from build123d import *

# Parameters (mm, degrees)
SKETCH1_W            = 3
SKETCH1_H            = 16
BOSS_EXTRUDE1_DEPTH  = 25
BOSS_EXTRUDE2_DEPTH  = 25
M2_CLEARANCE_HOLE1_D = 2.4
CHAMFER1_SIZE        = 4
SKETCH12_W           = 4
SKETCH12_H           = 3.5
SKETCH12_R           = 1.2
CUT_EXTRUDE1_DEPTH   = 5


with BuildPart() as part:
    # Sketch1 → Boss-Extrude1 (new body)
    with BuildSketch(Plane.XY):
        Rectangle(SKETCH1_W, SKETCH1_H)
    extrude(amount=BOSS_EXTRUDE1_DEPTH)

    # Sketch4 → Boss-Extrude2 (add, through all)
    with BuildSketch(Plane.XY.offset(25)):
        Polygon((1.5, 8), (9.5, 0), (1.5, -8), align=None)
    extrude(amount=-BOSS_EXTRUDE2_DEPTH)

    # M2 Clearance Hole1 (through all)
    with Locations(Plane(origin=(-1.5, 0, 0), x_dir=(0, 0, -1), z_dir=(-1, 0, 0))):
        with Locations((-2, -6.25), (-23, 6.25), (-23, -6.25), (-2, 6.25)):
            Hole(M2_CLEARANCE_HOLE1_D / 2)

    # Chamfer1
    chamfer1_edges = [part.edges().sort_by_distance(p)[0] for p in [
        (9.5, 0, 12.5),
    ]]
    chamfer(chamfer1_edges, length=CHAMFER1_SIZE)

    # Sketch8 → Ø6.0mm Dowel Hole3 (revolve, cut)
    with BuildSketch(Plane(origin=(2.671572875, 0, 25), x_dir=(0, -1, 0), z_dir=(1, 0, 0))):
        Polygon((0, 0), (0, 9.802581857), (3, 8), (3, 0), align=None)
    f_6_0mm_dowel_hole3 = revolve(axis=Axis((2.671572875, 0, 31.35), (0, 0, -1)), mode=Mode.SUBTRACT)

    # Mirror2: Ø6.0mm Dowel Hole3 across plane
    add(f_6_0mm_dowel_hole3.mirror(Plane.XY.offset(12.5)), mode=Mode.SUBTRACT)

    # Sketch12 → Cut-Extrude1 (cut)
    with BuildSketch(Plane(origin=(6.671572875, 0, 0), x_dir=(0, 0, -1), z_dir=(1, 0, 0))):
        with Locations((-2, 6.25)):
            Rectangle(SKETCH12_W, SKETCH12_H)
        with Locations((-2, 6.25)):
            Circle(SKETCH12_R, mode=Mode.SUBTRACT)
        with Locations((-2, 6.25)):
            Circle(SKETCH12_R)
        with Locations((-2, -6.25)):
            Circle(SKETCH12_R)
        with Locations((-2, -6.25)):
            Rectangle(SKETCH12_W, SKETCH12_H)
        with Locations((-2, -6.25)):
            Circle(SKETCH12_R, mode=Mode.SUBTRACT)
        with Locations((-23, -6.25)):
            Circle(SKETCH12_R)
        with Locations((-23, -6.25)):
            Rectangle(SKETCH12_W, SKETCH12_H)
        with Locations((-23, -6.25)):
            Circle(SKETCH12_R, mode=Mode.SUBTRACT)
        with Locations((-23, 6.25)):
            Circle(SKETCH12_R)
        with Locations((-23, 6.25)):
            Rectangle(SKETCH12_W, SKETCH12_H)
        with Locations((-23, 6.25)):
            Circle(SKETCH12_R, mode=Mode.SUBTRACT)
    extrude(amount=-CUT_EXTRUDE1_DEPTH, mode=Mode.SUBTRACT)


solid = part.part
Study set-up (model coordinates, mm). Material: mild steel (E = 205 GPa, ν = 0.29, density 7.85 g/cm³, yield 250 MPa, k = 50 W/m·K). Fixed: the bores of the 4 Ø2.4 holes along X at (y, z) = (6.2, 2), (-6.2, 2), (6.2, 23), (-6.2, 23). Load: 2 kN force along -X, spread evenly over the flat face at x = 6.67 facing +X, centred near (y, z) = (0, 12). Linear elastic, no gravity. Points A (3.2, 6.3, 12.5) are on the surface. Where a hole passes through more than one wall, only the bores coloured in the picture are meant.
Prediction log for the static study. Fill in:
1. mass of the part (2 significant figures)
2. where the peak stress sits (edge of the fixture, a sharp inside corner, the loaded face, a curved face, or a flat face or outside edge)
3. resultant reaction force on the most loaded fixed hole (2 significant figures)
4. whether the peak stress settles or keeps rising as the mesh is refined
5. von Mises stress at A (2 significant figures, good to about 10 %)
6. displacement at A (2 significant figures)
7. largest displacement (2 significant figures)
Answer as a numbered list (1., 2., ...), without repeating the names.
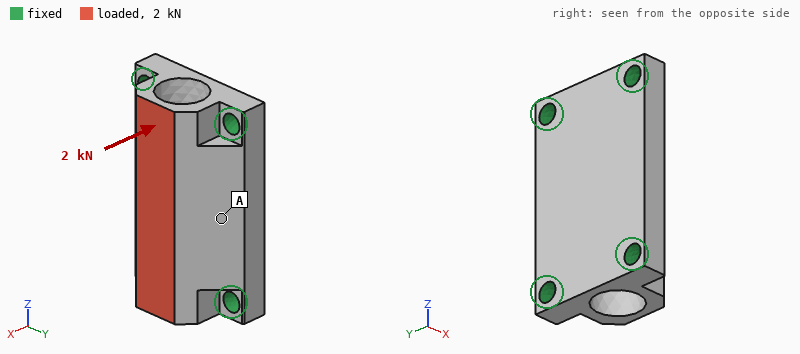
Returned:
1. 15 g
2. edge of the fixture
3. 550 N
4. keeps rising
5. 18 MPa
6. 2.2 µm
7. 3.0 µm
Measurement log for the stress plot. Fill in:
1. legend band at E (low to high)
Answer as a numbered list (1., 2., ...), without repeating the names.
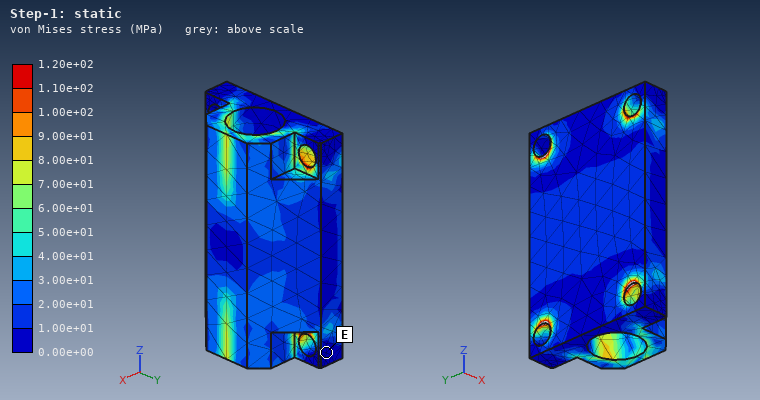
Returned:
1. 0.00e+00 to 1.00e+01 MPa
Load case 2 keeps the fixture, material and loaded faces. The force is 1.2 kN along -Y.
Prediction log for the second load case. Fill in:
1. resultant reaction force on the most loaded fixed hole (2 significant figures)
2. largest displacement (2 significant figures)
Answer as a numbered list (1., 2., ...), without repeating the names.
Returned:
1. 460 N
2. 3.6 µm
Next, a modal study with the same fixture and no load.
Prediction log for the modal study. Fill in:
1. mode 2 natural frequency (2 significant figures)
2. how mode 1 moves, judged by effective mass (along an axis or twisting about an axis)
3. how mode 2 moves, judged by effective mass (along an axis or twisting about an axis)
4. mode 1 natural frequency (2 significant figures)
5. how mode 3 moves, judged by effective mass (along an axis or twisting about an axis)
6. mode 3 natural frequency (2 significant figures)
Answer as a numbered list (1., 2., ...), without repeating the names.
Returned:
1. 43 kHz
2. along X
3. along Y
4. 39 kHz
5. along Y
6. 55 kHz
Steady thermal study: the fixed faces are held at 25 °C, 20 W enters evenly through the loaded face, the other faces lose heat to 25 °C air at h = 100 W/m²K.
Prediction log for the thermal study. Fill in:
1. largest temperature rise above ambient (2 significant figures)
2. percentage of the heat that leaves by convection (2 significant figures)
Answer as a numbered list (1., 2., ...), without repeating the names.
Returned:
1. 35 K
2. 10 %
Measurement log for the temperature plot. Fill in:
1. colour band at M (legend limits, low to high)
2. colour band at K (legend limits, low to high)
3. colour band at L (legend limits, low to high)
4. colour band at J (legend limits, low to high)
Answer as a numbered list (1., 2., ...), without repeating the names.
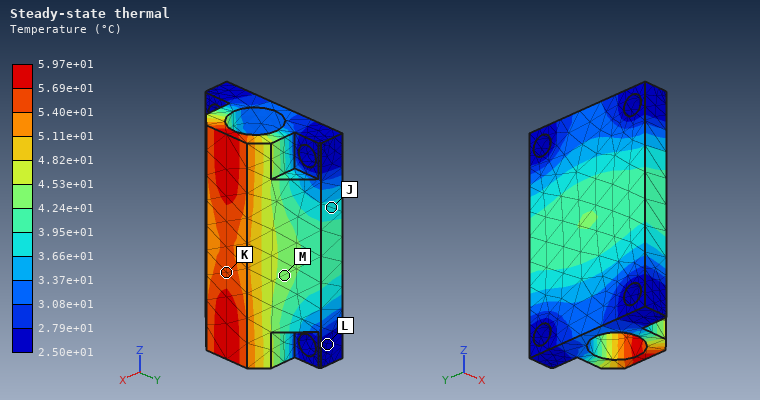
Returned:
1. 4.24e+01 to 4.53e+01 °C
2. 5.40e+01 to 5.69e+01 °C
3. 2.50e+01 to 2.79e+01 °C
4. 3.66e+01 to 3.95e+01 °C
